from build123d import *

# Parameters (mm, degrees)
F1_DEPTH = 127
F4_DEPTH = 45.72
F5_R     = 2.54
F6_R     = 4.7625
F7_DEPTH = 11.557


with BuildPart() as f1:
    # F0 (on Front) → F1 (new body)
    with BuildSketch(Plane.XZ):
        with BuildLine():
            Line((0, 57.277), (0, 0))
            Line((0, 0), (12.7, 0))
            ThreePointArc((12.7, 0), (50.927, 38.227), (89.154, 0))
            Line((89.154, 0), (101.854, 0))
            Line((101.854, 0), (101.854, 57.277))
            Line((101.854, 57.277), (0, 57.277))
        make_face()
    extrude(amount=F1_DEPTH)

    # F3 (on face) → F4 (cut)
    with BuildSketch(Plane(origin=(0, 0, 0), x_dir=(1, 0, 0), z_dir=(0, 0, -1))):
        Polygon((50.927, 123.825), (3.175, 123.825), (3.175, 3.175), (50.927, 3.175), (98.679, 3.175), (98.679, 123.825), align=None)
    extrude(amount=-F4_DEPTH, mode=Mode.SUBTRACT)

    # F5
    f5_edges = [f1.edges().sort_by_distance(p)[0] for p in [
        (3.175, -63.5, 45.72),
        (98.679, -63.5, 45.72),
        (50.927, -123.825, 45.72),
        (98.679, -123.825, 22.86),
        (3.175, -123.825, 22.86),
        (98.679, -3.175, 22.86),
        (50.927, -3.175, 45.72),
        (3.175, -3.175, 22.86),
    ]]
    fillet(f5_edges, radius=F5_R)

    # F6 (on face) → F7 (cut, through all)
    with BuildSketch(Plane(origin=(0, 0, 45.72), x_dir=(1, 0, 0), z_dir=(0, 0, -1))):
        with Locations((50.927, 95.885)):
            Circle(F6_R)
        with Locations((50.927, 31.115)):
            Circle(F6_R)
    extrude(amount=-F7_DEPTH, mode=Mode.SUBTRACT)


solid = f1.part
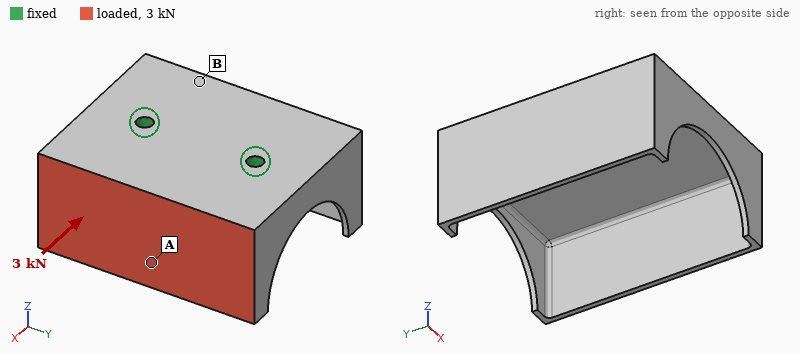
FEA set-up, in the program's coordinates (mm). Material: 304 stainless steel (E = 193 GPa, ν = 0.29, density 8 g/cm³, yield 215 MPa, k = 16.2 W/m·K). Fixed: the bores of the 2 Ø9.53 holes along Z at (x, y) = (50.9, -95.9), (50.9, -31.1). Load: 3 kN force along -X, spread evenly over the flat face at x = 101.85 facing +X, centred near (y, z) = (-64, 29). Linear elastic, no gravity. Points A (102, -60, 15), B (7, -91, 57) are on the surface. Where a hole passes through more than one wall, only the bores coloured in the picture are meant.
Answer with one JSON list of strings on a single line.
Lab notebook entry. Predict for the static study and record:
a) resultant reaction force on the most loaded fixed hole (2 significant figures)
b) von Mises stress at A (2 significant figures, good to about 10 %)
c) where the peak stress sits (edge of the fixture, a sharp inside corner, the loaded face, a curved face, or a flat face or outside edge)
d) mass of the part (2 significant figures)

["1.5 kN", "29 MPa", "a curved face", "1.6 kg"]
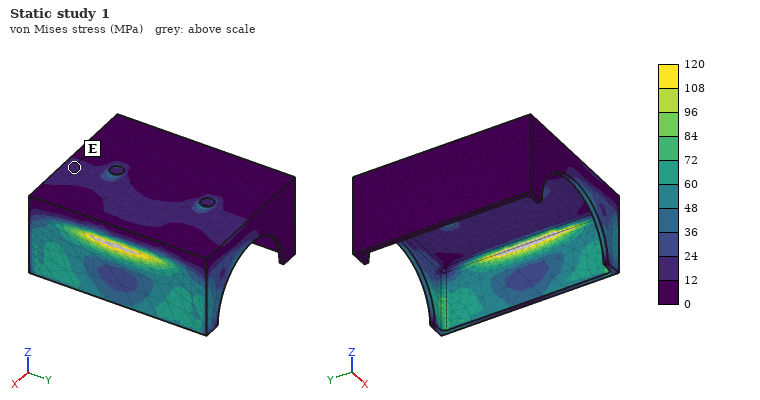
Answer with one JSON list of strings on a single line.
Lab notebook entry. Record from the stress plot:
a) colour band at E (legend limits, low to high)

["12 to 24 MPa"]
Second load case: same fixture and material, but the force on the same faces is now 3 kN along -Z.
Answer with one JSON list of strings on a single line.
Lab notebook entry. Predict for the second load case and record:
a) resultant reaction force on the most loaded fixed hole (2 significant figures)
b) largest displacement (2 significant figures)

["1.5 kN", "92 µm"]
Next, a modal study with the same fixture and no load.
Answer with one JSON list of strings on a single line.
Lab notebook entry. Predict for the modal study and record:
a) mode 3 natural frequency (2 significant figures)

["2100 Hz"]
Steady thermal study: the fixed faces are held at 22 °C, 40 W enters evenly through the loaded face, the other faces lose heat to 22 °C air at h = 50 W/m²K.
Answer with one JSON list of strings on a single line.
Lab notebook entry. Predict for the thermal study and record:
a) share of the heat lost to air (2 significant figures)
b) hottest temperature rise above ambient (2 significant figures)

["79 %", "66 K"]
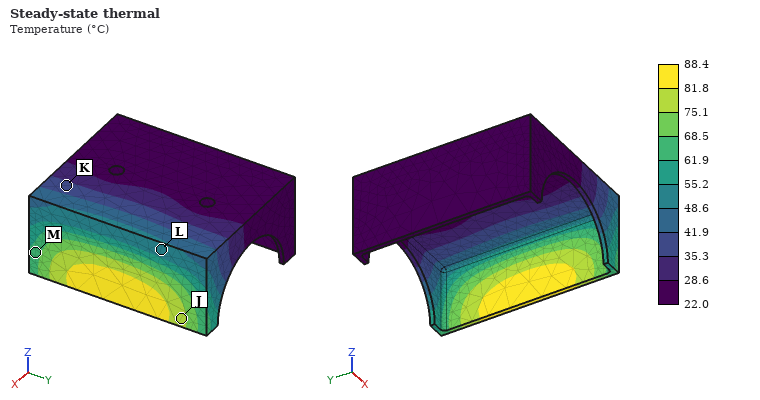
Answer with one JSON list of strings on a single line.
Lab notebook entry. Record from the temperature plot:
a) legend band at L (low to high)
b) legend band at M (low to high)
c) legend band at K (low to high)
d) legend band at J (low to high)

["48.6 to 55.2 °C", "61.9 to 68.5 °C", "35.3 to 41.9 °C", "75.1 to 81.8 °C"]
